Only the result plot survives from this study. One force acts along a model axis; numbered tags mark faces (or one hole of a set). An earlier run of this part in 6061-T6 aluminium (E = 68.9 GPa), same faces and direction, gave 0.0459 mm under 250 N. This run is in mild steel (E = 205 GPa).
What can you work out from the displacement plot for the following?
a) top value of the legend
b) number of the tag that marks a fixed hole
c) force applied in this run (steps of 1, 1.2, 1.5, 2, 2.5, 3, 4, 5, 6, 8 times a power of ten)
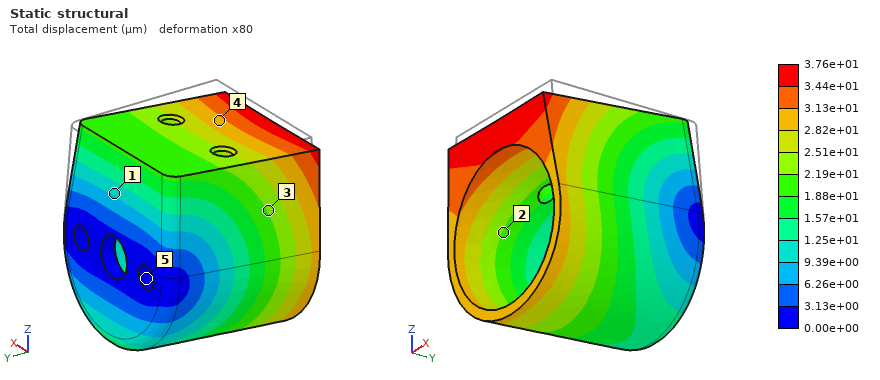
3.76e+01 µm
5
600 N
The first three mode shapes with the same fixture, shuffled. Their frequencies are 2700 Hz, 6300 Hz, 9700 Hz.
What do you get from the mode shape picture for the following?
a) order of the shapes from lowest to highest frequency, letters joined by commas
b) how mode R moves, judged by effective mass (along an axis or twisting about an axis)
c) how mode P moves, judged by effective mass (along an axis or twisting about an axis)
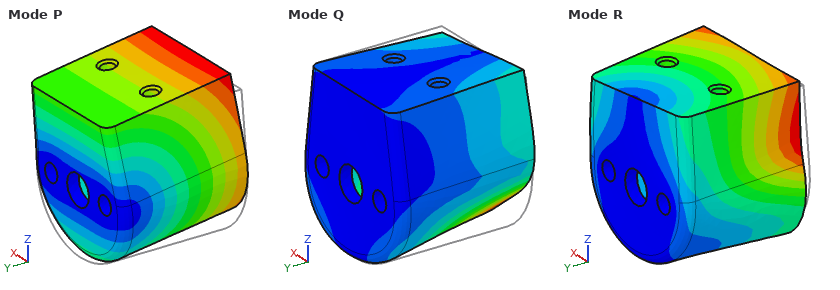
P, R, Q
along X
along Z
